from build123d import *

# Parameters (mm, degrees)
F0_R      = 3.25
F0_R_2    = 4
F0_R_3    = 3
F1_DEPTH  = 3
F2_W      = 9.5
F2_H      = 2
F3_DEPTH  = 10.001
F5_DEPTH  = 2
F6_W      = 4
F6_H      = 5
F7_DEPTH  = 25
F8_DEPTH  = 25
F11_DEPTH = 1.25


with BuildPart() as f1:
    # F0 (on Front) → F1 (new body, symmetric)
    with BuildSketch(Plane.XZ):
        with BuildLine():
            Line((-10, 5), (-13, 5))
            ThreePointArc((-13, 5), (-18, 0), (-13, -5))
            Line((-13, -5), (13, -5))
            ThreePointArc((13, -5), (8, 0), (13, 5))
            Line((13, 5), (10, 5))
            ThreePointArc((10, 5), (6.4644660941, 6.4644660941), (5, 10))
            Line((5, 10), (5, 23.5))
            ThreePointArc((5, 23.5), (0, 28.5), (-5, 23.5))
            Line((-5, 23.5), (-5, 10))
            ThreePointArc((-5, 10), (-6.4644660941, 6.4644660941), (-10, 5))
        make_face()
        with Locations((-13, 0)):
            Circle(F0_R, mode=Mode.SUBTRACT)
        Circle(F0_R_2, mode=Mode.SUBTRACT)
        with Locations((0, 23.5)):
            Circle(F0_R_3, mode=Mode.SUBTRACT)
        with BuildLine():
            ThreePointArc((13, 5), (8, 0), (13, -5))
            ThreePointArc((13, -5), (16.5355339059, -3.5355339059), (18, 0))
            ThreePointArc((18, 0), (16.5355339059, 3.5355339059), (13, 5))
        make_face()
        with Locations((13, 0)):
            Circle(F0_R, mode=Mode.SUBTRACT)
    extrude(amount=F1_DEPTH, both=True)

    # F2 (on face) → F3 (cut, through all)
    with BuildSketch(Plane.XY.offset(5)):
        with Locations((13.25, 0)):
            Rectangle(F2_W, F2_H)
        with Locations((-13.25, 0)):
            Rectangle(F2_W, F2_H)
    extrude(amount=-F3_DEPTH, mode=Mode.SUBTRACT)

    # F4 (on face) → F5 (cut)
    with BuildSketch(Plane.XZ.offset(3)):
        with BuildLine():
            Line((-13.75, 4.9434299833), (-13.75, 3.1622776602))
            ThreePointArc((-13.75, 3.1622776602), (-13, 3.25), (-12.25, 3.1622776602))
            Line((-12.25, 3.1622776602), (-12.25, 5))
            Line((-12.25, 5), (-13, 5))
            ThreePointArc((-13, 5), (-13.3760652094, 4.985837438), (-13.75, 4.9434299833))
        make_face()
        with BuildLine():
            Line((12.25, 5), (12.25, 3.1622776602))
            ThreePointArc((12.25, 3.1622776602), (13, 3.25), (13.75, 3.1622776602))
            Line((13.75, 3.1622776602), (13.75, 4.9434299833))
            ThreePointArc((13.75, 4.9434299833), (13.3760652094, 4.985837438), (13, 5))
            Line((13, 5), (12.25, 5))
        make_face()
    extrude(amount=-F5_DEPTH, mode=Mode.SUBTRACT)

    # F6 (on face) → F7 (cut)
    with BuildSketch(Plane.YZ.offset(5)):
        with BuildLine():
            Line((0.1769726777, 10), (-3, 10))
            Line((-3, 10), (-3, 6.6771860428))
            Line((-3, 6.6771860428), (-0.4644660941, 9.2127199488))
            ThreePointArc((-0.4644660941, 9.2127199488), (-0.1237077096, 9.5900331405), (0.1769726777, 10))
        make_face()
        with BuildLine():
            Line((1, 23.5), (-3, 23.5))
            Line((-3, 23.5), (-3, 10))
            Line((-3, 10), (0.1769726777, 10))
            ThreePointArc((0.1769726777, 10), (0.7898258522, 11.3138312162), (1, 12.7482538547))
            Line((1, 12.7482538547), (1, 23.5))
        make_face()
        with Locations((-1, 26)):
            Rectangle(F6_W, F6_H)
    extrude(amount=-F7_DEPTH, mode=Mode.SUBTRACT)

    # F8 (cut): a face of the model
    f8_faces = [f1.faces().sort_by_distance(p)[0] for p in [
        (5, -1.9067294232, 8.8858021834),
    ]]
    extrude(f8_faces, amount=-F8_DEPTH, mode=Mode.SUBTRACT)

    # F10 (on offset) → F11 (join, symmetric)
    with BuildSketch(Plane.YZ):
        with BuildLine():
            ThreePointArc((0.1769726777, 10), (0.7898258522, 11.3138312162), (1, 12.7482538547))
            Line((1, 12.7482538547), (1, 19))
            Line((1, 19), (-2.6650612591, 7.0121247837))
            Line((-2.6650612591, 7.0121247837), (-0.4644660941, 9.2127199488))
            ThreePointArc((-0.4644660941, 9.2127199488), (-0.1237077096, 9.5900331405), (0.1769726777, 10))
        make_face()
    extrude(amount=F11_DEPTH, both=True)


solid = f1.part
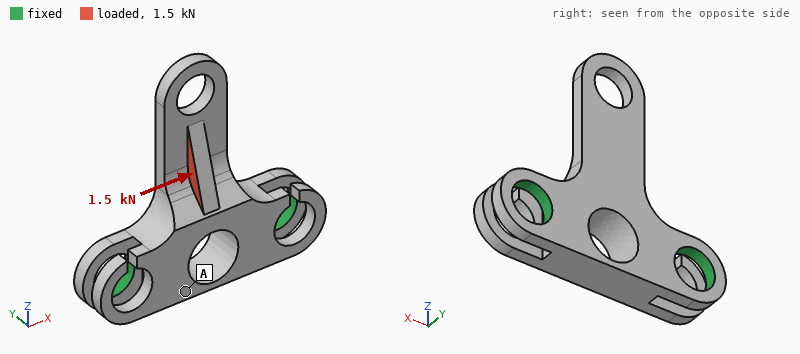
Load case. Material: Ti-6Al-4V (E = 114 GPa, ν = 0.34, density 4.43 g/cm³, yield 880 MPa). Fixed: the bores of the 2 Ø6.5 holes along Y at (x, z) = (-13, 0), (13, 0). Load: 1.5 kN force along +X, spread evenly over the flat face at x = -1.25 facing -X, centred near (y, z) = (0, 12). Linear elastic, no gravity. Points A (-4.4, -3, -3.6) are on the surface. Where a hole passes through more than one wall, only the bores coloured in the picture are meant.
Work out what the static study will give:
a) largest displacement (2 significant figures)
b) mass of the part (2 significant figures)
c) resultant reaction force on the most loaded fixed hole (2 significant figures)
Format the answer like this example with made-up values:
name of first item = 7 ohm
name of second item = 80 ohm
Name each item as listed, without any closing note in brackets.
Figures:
largest displacement = 56 µm
mass of the part = 7.8 g
resultant reaction force on the most loaded fixed hole = 1.2 kN
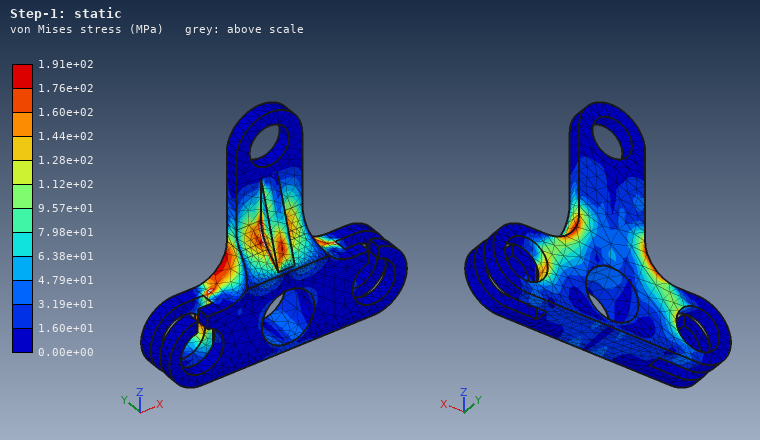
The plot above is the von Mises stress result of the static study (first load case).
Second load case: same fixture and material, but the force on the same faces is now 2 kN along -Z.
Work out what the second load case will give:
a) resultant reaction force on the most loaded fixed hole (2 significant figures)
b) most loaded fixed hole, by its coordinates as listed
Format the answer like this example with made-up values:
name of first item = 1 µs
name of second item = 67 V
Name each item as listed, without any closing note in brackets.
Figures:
resultant reaction force on the most loaded fixed hole = 1.2 kN
most loaded fixed hole, by its coordinates as listed = (-13, 0)
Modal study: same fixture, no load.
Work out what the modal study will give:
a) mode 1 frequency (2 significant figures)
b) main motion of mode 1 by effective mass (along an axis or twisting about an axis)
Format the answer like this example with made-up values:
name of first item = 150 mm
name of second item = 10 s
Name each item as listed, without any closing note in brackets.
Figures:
mode 1 frequency = 5800 Hz
main motion of mode 1 by effective mass = along Y
